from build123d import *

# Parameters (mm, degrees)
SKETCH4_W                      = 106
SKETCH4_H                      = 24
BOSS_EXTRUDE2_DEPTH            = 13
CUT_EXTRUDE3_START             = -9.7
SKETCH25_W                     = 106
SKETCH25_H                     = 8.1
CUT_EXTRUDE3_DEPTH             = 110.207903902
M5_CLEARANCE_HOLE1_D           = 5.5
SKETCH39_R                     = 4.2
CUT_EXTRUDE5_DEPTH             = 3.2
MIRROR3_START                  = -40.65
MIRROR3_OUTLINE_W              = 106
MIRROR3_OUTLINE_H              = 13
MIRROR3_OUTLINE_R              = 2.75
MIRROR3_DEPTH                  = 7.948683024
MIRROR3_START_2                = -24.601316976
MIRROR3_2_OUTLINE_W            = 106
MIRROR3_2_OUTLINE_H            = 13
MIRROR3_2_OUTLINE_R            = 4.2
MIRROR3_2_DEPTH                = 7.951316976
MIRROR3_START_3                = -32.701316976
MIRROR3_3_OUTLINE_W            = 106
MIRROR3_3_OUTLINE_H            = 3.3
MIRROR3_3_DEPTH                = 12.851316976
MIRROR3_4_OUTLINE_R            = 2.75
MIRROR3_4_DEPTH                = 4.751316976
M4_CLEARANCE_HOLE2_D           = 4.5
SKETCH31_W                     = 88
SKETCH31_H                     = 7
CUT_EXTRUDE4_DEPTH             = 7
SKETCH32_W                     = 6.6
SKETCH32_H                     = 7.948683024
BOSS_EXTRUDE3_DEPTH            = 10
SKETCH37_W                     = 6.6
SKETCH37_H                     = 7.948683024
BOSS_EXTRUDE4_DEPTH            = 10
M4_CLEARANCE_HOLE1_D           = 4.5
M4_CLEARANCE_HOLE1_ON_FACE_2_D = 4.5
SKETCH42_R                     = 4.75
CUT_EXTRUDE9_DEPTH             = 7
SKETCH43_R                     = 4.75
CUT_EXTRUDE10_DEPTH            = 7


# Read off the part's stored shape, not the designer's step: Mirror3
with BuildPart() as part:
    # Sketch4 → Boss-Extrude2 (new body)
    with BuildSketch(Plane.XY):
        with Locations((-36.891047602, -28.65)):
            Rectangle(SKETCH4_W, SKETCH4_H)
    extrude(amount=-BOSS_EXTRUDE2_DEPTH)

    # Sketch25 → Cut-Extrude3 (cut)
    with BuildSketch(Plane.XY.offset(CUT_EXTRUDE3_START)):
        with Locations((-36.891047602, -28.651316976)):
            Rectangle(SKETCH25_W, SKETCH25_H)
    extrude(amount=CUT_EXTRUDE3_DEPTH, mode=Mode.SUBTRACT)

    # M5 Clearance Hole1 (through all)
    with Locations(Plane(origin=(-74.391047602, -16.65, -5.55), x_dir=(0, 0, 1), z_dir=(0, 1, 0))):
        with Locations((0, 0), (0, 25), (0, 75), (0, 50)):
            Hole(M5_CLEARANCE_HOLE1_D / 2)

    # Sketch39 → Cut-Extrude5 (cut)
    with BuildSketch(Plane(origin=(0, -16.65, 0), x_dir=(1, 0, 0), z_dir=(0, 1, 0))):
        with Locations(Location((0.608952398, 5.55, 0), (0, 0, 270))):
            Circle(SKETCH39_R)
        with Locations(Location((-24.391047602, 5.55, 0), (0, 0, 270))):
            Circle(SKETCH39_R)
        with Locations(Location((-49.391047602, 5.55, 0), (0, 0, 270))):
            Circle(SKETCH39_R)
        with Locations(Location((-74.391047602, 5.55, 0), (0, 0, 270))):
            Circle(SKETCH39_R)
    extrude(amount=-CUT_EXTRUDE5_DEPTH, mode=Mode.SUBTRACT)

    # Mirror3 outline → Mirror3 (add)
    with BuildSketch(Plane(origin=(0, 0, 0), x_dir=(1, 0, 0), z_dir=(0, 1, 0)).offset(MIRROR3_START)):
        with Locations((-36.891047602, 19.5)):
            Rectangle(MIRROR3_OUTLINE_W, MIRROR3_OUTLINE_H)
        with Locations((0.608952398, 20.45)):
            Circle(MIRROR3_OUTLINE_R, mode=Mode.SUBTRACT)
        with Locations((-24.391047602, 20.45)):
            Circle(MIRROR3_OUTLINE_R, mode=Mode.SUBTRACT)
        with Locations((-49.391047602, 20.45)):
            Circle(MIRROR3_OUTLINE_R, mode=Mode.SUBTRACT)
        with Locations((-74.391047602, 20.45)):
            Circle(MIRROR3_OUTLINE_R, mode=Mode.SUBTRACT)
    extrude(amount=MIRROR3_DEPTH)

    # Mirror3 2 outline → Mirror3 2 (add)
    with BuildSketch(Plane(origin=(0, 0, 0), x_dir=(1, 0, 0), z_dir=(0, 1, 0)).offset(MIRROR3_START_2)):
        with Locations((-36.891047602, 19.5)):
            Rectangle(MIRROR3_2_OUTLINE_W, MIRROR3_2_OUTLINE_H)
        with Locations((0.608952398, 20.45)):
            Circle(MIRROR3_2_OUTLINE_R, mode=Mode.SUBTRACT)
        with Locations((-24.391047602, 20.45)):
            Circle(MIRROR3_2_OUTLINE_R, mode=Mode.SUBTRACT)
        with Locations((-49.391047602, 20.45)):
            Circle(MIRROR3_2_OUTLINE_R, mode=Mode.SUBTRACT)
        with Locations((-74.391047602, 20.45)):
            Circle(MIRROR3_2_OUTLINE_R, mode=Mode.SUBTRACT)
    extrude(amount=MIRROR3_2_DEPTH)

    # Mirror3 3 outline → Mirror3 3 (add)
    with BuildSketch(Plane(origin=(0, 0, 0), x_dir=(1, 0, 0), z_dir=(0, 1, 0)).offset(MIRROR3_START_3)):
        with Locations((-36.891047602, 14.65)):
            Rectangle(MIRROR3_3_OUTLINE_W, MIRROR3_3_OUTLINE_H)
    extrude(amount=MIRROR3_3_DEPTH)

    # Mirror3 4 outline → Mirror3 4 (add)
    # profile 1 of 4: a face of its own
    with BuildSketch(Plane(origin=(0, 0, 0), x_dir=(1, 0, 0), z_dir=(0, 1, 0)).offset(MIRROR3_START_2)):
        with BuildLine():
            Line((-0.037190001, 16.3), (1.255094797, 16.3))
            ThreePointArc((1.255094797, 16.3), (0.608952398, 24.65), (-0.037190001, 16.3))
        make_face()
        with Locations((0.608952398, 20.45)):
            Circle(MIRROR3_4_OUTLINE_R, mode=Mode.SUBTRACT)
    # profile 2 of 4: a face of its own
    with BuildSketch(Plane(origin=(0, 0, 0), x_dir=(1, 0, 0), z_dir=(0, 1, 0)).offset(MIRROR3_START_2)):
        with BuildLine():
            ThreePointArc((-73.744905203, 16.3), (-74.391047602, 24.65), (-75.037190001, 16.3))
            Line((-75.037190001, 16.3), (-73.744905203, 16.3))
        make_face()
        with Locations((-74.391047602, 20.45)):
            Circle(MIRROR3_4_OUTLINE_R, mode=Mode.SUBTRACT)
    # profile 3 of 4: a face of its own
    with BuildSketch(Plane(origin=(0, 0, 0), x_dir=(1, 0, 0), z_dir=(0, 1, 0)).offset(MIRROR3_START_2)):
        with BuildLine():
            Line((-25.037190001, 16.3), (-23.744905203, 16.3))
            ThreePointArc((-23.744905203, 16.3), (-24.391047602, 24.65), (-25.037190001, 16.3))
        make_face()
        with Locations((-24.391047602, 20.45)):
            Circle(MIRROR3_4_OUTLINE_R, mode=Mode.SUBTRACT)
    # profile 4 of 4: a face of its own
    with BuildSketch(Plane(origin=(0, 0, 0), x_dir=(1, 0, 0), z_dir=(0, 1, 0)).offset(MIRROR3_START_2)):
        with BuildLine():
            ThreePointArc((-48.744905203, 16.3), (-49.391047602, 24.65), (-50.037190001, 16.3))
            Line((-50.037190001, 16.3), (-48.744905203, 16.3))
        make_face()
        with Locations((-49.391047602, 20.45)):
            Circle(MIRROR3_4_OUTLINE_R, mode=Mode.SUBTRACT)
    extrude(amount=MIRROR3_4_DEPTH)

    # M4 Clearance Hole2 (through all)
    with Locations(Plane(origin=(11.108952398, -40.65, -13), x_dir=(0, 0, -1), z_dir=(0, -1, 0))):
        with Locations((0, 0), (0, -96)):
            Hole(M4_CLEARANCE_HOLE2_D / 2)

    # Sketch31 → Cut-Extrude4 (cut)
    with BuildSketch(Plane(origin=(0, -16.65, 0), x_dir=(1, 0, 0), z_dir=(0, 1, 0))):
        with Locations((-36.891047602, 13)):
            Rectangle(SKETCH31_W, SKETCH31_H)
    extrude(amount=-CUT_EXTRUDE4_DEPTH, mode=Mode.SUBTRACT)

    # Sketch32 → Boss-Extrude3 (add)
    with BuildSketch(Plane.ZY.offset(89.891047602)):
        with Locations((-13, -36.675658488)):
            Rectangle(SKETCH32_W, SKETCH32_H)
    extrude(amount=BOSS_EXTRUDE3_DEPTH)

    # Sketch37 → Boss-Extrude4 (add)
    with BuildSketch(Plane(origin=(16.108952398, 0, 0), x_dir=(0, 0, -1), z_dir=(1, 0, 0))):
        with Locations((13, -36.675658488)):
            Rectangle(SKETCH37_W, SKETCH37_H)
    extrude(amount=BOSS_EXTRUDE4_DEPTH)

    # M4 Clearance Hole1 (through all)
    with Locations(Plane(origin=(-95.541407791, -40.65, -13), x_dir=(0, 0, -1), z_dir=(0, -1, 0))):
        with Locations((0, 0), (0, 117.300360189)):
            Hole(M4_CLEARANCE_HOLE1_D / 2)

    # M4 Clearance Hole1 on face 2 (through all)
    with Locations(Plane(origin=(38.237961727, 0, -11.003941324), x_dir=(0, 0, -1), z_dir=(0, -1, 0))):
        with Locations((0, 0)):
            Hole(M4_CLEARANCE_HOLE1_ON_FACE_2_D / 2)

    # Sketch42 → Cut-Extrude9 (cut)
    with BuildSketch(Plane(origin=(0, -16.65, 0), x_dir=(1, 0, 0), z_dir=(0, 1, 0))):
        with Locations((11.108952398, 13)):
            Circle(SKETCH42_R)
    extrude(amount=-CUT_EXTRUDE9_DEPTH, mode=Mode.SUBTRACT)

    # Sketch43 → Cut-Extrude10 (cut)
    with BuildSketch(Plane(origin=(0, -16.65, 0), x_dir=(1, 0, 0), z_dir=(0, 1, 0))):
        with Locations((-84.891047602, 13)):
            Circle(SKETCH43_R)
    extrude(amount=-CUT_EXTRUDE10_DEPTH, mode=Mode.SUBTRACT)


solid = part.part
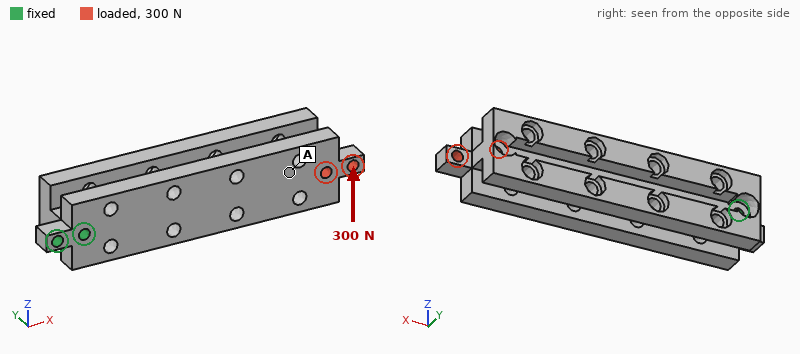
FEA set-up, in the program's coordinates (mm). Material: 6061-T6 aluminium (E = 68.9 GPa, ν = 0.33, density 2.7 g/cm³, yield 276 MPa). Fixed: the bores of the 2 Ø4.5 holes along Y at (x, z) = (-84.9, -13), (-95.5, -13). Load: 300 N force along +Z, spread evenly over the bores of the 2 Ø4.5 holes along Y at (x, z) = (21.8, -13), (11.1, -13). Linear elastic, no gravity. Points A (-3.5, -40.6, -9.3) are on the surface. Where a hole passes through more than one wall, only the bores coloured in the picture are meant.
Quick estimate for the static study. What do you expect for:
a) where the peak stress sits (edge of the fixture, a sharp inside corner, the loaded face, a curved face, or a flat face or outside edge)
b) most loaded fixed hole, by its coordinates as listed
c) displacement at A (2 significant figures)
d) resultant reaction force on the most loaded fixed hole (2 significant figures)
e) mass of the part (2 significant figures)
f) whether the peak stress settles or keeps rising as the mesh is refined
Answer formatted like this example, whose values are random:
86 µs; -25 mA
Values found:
edge of the fixture; (-84.9, -13); 0.17 mm; 1.1 kN; 110 g; keeps rising
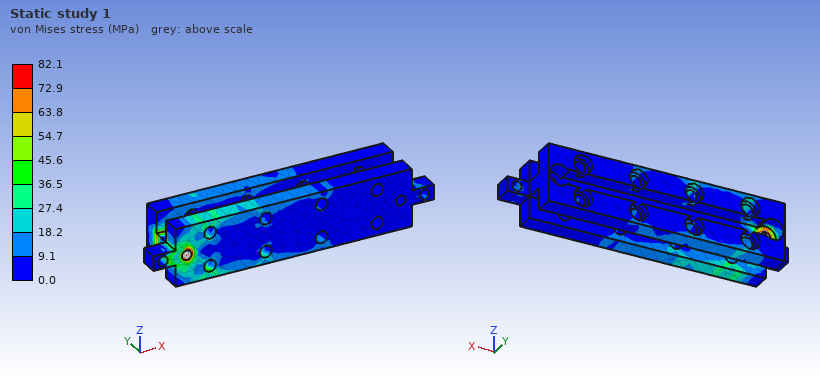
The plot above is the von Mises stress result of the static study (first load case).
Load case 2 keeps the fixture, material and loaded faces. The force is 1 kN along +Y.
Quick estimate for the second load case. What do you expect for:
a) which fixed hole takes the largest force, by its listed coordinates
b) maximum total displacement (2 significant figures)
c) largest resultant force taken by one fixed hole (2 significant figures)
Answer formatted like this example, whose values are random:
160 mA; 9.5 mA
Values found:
(-84.9, -13); 0.62 mm; 1.4 kN
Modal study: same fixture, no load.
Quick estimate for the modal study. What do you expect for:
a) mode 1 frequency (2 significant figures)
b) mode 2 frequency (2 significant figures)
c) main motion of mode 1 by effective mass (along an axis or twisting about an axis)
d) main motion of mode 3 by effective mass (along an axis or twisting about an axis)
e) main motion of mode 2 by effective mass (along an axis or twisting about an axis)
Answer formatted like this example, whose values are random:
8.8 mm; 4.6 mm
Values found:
1000 Hz; 1300 Hz; along Z; twisting about X; along Y
